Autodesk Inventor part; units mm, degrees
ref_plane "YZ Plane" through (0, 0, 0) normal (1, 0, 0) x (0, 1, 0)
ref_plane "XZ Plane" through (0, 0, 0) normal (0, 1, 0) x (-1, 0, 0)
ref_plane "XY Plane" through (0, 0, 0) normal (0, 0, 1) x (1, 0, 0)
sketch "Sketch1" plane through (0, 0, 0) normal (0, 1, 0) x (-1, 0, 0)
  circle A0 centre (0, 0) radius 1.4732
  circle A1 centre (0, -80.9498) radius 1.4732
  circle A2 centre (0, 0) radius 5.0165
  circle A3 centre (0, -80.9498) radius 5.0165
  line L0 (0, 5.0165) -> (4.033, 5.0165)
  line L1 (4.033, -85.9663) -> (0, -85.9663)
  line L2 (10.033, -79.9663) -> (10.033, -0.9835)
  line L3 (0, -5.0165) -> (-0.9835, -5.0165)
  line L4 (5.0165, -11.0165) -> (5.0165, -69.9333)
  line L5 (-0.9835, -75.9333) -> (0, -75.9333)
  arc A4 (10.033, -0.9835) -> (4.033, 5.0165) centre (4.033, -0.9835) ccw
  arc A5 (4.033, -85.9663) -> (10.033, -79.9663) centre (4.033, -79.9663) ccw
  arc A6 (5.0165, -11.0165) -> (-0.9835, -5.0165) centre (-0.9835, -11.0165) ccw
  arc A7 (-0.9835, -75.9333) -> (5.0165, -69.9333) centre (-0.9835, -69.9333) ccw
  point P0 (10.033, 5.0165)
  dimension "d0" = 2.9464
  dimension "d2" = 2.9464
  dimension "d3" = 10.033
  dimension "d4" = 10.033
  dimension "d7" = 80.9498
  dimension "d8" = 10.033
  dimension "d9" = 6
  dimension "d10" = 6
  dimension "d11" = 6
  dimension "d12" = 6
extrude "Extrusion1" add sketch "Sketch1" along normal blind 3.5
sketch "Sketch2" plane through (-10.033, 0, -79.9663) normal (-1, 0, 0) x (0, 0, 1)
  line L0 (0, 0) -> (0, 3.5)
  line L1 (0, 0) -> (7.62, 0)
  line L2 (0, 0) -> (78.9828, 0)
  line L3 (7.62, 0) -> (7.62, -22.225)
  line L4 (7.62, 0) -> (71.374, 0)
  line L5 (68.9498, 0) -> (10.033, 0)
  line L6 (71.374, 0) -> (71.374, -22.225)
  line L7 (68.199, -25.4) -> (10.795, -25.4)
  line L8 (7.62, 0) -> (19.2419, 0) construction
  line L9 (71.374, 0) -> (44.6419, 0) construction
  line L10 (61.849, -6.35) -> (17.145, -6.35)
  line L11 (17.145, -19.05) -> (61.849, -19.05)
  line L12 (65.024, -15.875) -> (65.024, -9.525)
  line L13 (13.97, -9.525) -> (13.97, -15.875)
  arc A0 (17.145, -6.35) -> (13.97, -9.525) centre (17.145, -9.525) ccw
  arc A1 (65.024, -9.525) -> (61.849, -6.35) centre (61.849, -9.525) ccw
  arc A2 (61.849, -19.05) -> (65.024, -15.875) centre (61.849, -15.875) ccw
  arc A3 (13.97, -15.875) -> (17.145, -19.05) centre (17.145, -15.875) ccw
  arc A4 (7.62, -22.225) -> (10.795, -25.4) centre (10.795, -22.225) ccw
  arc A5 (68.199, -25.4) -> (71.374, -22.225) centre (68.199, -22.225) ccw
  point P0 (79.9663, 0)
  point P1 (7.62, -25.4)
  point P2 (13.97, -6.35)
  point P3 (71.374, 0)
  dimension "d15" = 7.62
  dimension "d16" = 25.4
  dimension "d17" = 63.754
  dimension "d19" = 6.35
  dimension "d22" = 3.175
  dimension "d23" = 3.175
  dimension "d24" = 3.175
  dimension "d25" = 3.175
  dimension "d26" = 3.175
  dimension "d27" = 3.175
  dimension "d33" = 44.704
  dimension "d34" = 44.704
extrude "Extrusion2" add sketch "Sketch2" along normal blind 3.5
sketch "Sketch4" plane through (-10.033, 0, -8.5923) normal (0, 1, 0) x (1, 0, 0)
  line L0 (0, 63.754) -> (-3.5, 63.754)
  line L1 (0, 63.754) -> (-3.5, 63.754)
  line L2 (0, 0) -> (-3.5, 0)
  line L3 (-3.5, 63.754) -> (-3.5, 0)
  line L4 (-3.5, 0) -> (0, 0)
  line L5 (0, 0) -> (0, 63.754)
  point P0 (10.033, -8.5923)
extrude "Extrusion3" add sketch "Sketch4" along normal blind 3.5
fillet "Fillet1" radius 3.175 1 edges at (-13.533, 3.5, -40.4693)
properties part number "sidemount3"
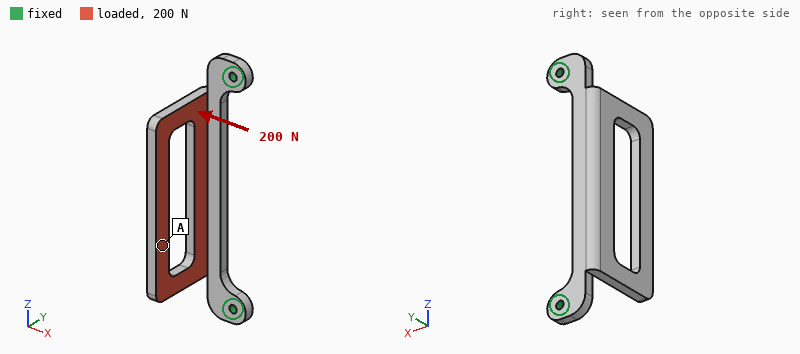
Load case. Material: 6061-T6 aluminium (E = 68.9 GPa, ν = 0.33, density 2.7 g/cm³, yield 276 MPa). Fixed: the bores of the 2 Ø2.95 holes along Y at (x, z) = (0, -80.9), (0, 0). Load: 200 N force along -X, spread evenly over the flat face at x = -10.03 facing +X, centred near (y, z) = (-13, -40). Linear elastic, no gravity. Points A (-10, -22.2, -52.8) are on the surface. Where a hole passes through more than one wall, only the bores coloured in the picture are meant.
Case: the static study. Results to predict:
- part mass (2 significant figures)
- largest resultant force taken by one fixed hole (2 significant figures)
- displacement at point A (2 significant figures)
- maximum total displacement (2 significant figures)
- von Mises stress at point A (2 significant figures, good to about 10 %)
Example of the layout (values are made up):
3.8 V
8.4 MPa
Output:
17 g
160 N
0.45 mm
0.53 mm
18 MPa
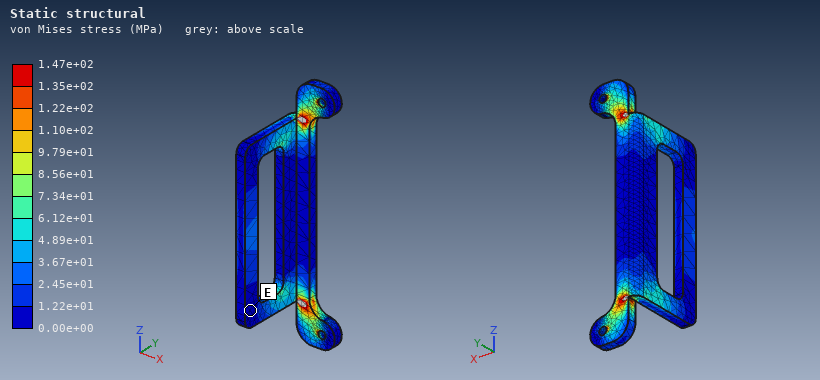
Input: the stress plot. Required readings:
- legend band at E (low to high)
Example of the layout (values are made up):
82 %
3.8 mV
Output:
0.00e+00 to 1.22e+01 MPa
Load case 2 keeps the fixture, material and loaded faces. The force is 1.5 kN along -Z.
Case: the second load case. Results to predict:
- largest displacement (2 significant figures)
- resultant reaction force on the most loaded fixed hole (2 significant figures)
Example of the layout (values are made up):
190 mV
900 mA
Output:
0.27 mm
810 N
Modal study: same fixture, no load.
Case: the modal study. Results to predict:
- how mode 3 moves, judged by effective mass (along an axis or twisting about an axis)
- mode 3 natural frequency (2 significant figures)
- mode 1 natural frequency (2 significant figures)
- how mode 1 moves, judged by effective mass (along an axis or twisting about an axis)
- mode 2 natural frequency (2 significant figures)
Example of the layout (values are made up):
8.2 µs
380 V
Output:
along Y
3400 Hz
1200 Hz
along X
3100 Hz
